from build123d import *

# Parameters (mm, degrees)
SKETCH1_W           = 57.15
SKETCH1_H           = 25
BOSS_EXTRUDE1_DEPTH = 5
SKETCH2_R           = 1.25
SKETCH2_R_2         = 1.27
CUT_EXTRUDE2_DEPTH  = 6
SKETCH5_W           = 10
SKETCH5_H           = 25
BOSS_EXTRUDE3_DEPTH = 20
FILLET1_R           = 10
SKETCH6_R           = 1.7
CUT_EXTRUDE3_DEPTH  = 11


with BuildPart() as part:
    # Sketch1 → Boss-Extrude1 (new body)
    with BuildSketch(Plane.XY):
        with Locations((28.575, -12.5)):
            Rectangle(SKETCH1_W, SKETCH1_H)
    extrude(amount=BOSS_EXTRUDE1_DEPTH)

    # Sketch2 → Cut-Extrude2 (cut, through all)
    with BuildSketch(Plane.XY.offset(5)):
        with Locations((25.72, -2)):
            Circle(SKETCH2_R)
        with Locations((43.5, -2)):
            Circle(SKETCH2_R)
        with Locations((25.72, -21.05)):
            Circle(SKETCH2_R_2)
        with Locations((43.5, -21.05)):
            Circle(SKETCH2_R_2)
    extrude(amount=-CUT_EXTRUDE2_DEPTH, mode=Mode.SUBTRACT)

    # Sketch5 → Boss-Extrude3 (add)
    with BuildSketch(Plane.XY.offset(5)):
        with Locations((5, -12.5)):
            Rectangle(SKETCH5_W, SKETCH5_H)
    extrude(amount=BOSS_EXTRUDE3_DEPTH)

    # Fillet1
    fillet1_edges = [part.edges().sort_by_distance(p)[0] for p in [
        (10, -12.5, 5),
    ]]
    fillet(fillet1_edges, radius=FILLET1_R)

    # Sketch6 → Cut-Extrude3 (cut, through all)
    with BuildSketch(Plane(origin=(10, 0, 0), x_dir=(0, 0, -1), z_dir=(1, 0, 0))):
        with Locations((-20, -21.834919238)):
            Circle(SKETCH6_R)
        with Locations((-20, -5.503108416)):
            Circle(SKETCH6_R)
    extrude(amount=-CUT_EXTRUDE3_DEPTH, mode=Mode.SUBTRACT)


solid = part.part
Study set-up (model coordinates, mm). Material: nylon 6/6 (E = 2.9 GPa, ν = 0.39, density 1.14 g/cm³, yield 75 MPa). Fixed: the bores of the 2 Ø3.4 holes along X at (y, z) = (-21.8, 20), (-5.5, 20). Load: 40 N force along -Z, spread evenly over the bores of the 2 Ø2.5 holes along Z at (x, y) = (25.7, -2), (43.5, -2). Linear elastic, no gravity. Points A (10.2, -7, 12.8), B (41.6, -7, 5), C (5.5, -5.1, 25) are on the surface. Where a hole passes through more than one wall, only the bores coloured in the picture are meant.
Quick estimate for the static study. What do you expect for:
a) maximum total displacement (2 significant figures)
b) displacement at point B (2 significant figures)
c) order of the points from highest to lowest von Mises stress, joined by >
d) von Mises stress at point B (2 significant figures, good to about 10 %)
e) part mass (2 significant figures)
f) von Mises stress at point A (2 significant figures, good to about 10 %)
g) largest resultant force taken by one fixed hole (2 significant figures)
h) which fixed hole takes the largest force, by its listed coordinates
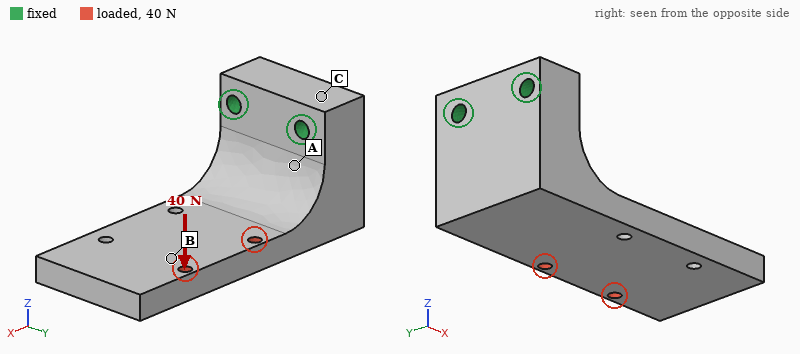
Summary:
0.71 mm
0.39 mm
A > B > C
1.7 MPa
14 g
4.1 MPa
47 N
(-5.5, 20)
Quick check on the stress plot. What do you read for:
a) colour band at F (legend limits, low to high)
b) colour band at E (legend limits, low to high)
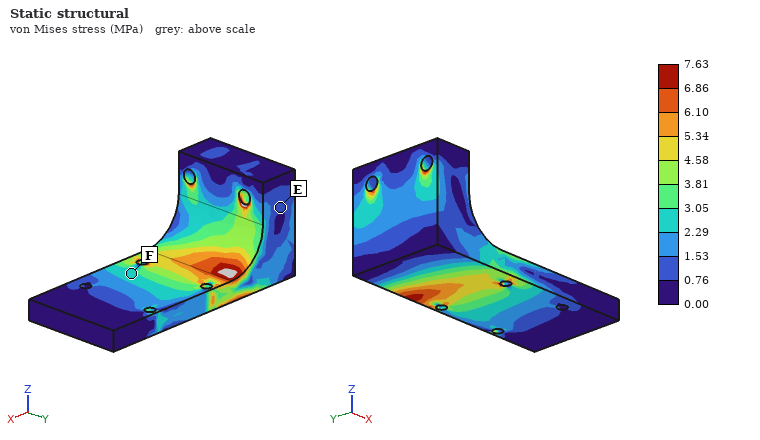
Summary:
2.29 to 3.05 MPa
0.76 to 1.53 MPa
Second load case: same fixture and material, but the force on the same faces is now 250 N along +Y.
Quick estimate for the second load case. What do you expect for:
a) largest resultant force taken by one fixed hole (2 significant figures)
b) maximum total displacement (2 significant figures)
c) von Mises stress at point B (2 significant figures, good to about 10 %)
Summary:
440 N
0.80 mm
3.2 MPa
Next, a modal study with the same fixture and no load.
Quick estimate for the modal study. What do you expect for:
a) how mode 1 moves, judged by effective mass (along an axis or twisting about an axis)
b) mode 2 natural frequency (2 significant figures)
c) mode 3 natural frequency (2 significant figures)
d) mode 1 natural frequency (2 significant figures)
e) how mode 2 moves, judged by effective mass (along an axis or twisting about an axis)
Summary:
along Z
1300 Hz
2200 Hz
600 Hz
along Y
